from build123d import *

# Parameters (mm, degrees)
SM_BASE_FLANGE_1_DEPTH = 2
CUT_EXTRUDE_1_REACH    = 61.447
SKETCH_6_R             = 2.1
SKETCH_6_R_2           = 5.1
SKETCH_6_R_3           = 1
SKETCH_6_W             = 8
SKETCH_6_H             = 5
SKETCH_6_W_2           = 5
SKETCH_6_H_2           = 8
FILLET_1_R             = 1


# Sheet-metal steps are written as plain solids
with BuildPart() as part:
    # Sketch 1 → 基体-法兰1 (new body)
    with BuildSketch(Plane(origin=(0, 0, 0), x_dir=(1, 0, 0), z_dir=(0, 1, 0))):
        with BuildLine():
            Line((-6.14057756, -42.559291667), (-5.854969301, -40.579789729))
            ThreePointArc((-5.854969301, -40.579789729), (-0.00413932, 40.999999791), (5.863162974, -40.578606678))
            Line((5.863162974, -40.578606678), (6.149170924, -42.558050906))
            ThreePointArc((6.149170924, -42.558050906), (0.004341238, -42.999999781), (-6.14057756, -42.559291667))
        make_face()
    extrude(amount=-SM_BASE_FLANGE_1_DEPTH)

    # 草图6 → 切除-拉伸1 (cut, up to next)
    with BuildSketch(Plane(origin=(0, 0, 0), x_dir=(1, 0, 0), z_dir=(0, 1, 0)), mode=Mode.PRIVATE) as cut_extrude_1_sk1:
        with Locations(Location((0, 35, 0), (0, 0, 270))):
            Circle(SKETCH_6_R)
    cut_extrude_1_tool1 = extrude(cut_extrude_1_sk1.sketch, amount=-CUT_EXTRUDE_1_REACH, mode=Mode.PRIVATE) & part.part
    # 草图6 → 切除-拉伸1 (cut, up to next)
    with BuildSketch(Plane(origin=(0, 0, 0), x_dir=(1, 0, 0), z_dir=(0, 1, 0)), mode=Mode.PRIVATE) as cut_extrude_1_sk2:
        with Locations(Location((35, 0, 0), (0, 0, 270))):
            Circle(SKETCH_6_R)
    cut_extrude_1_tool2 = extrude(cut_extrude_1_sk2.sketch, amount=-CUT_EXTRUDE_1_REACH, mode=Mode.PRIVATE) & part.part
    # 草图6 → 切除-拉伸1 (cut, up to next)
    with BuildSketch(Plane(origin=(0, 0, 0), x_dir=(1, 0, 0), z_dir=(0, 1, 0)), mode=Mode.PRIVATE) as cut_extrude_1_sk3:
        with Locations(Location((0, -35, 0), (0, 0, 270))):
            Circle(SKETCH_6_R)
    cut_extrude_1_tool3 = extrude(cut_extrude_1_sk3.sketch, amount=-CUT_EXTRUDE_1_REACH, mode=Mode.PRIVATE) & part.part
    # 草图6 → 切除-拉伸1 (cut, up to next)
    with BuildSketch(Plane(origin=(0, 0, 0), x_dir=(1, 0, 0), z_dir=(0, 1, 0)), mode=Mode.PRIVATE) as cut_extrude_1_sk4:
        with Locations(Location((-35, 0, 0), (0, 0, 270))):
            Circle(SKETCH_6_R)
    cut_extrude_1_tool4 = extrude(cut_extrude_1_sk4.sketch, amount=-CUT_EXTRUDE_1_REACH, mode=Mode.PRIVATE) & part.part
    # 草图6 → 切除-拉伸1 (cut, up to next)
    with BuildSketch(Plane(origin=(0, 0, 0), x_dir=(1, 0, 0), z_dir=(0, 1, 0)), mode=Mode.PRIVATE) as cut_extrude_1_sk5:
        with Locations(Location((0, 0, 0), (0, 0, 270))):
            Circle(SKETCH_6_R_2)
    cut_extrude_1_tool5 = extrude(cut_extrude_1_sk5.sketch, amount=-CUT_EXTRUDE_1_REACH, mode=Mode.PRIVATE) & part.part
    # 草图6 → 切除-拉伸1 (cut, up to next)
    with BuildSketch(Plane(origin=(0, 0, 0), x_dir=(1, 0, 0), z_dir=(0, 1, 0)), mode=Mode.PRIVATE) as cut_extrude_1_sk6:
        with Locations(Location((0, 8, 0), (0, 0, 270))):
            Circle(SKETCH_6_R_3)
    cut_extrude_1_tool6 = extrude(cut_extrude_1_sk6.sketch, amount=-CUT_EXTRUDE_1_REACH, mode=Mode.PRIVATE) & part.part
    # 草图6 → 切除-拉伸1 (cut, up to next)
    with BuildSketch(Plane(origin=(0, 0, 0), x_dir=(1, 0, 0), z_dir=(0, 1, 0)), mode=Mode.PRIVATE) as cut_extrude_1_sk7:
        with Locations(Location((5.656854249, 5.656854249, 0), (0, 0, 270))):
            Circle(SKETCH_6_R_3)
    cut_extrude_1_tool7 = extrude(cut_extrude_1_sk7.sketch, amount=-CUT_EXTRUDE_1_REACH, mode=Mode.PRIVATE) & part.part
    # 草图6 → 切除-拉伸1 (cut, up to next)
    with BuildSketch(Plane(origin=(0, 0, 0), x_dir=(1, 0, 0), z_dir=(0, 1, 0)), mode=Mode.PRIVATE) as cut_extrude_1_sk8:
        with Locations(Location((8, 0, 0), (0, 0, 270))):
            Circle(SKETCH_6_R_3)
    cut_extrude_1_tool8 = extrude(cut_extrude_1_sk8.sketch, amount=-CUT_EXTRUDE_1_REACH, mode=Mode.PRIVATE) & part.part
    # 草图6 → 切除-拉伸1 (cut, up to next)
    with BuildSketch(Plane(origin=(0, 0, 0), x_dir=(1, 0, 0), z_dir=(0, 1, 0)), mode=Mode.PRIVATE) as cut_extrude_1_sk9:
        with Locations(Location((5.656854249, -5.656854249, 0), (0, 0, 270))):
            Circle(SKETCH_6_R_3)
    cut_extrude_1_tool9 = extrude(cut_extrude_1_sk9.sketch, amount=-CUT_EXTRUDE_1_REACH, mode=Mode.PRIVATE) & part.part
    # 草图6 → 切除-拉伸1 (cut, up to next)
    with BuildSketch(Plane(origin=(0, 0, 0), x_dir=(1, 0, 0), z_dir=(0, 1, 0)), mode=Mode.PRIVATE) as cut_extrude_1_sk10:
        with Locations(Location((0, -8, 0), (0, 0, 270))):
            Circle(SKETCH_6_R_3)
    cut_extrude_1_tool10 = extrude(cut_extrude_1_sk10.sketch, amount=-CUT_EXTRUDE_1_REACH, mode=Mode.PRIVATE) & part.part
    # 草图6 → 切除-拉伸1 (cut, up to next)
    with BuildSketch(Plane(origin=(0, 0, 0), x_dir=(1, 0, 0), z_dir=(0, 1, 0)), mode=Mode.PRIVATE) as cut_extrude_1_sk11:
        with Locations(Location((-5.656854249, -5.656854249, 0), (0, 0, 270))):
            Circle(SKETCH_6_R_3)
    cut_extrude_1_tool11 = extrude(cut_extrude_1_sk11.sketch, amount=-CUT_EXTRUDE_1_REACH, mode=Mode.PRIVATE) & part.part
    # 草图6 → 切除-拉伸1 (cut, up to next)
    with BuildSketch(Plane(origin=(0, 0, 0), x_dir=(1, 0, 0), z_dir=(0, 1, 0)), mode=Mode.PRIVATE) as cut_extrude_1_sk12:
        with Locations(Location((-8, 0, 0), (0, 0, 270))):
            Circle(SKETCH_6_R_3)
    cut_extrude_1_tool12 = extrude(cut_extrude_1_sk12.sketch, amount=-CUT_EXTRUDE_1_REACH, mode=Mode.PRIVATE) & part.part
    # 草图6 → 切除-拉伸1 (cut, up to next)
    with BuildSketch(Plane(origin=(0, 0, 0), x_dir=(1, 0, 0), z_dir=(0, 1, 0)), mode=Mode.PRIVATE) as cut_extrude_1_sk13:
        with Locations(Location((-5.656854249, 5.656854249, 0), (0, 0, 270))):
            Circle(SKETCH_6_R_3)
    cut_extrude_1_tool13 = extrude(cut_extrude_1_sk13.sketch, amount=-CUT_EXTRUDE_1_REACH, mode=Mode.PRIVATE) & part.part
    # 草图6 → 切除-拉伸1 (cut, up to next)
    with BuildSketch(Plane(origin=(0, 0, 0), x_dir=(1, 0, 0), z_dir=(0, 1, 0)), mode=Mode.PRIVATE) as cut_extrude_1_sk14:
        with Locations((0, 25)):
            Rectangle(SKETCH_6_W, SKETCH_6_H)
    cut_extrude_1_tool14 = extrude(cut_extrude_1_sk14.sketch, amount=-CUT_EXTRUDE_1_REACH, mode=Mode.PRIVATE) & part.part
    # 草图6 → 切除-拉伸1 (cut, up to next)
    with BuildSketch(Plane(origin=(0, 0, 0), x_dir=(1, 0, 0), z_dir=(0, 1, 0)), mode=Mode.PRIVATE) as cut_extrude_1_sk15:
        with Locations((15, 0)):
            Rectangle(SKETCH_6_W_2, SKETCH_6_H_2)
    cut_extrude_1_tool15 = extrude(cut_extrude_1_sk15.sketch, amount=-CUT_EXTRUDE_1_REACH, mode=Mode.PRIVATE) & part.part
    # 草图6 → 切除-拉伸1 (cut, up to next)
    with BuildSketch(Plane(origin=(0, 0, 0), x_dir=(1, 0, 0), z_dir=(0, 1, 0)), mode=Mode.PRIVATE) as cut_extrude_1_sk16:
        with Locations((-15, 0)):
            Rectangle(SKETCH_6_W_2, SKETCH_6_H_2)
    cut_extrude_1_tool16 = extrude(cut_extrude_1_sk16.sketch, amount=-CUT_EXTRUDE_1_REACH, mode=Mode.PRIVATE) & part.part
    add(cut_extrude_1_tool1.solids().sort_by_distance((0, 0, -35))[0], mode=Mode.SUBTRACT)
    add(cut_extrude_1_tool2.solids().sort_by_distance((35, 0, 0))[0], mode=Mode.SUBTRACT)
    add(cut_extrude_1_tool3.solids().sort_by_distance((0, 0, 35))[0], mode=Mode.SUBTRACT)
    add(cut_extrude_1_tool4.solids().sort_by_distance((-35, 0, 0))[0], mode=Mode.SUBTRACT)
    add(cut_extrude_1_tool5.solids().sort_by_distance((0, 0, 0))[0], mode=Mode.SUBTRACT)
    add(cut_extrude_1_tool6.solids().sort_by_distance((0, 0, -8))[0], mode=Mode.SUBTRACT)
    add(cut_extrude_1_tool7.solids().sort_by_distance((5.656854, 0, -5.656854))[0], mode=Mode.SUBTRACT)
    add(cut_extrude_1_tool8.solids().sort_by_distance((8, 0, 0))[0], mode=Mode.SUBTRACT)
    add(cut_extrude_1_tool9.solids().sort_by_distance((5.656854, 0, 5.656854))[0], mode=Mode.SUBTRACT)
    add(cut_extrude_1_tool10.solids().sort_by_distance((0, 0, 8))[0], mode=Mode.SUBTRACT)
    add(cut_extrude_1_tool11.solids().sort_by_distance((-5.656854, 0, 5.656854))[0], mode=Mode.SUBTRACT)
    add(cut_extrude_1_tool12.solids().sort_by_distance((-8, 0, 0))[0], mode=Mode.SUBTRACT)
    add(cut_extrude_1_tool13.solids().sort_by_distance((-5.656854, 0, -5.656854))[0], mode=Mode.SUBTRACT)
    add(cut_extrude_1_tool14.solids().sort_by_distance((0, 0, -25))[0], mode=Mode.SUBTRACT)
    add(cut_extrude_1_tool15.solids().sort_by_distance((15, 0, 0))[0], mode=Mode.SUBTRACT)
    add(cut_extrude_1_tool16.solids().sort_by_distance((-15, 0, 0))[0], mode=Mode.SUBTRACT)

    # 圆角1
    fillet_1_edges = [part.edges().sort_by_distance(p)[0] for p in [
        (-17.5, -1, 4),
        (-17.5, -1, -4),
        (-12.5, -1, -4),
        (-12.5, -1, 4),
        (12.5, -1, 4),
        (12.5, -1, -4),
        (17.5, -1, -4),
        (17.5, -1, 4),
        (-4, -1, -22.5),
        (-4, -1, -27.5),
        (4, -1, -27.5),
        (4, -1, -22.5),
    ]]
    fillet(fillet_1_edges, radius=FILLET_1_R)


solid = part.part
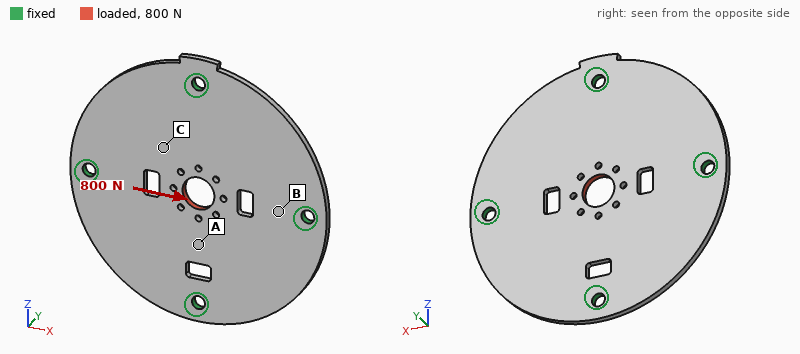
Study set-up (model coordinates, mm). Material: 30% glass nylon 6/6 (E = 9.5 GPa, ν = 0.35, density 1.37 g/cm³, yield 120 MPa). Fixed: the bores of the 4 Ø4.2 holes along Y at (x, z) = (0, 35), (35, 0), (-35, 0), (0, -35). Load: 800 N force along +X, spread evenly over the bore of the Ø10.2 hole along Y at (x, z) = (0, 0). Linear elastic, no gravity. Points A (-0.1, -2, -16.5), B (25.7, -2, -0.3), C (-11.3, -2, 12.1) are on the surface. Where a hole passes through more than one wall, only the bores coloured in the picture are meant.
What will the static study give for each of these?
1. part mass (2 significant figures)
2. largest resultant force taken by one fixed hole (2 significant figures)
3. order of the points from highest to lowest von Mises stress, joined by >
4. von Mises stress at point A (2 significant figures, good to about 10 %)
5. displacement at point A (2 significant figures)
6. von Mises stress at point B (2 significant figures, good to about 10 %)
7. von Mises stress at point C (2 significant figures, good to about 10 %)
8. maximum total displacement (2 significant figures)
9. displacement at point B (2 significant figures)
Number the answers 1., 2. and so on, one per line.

1. 14 g
2. 250 N
3. B > C > A
4. 2.1 MPa
5. 17 µm
6. 7.8 MPa
7. 4.1 MPa
8. 42 µm
9. 7.9 µm
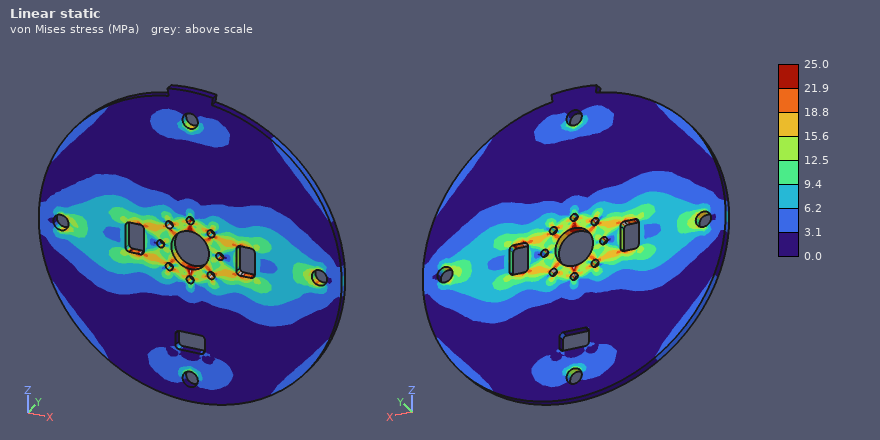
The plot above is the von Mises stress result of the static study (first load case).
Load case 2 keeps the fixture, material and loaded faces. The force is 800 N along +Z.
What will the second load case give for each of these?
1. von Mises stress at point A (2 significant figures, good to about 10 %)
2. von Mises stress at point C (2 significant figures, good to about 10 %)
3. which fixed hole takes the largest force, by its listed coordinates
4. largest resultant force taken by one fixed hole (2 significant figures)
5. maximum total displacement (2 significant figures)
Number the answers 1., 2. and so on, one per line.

1. 5.9 MPa
2. 5.4 MPa
3. (0, 35)
4. 290 N
5. 38 µm
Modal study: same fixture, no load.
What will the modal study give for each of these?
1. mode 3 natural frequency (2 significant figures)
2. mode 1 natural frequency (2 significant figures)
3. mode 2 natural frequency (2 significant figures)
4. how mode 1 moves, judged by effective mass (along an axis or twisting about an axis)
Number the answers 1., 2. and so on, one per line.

1. 1900 Hz
2. 1700 Hz
3. 1900 Hz
4. along Y
